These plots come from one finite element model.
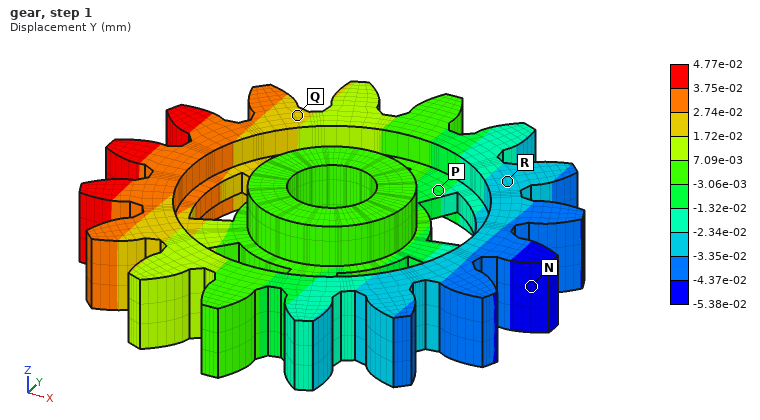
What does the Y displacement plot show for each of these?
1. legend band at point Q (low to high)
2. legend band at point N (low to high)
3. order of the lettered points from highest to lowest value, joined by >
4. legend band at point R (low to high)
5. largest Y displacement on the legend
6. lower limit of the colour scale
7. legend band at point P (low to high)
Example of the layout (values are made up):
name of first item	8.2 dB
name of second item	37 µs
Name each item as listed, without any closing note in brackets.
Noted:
legend band at point Q	1.72e-02 to 2.74e-02 mm
legend band at point N	-5.38e-02 to -4.37e-02 mm
order of the lettered points from highest to lowest value, joined by >	Q > P > R > N
legend band at point R	-3.35e-02 to -2.34e-02 mm
largest Y displacement on the legend	4.77e-02 mm
lower limit of the colour scale	-5.38e-02 mm
legend band at point P	-1.32e-02 to -3.06e-03 mm
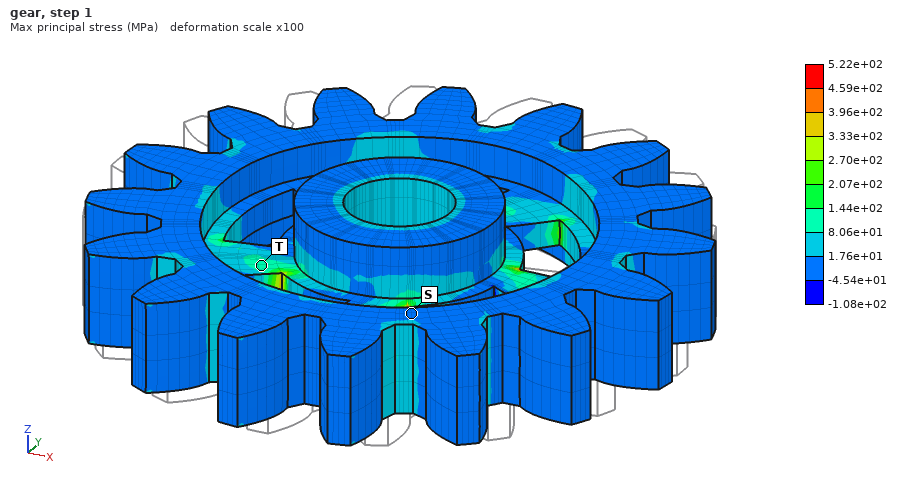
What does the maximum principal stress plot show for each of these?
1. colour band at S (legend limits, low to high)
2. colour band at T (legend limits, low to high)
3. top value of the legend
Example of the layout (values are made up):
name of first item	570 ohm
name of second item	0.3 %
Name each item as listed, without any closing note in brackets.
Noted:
colour band at S	-4.54e+01 to 1.76e+01 MPa
colour band at T	8.06e+01 to 1.44e+02 MPa
top value of the legend	5.22e+02 MPa
